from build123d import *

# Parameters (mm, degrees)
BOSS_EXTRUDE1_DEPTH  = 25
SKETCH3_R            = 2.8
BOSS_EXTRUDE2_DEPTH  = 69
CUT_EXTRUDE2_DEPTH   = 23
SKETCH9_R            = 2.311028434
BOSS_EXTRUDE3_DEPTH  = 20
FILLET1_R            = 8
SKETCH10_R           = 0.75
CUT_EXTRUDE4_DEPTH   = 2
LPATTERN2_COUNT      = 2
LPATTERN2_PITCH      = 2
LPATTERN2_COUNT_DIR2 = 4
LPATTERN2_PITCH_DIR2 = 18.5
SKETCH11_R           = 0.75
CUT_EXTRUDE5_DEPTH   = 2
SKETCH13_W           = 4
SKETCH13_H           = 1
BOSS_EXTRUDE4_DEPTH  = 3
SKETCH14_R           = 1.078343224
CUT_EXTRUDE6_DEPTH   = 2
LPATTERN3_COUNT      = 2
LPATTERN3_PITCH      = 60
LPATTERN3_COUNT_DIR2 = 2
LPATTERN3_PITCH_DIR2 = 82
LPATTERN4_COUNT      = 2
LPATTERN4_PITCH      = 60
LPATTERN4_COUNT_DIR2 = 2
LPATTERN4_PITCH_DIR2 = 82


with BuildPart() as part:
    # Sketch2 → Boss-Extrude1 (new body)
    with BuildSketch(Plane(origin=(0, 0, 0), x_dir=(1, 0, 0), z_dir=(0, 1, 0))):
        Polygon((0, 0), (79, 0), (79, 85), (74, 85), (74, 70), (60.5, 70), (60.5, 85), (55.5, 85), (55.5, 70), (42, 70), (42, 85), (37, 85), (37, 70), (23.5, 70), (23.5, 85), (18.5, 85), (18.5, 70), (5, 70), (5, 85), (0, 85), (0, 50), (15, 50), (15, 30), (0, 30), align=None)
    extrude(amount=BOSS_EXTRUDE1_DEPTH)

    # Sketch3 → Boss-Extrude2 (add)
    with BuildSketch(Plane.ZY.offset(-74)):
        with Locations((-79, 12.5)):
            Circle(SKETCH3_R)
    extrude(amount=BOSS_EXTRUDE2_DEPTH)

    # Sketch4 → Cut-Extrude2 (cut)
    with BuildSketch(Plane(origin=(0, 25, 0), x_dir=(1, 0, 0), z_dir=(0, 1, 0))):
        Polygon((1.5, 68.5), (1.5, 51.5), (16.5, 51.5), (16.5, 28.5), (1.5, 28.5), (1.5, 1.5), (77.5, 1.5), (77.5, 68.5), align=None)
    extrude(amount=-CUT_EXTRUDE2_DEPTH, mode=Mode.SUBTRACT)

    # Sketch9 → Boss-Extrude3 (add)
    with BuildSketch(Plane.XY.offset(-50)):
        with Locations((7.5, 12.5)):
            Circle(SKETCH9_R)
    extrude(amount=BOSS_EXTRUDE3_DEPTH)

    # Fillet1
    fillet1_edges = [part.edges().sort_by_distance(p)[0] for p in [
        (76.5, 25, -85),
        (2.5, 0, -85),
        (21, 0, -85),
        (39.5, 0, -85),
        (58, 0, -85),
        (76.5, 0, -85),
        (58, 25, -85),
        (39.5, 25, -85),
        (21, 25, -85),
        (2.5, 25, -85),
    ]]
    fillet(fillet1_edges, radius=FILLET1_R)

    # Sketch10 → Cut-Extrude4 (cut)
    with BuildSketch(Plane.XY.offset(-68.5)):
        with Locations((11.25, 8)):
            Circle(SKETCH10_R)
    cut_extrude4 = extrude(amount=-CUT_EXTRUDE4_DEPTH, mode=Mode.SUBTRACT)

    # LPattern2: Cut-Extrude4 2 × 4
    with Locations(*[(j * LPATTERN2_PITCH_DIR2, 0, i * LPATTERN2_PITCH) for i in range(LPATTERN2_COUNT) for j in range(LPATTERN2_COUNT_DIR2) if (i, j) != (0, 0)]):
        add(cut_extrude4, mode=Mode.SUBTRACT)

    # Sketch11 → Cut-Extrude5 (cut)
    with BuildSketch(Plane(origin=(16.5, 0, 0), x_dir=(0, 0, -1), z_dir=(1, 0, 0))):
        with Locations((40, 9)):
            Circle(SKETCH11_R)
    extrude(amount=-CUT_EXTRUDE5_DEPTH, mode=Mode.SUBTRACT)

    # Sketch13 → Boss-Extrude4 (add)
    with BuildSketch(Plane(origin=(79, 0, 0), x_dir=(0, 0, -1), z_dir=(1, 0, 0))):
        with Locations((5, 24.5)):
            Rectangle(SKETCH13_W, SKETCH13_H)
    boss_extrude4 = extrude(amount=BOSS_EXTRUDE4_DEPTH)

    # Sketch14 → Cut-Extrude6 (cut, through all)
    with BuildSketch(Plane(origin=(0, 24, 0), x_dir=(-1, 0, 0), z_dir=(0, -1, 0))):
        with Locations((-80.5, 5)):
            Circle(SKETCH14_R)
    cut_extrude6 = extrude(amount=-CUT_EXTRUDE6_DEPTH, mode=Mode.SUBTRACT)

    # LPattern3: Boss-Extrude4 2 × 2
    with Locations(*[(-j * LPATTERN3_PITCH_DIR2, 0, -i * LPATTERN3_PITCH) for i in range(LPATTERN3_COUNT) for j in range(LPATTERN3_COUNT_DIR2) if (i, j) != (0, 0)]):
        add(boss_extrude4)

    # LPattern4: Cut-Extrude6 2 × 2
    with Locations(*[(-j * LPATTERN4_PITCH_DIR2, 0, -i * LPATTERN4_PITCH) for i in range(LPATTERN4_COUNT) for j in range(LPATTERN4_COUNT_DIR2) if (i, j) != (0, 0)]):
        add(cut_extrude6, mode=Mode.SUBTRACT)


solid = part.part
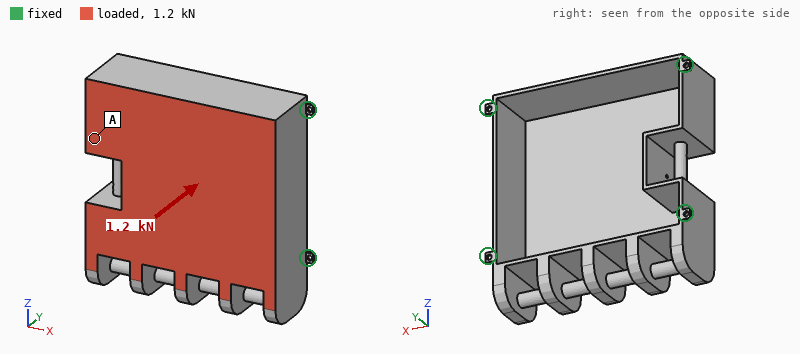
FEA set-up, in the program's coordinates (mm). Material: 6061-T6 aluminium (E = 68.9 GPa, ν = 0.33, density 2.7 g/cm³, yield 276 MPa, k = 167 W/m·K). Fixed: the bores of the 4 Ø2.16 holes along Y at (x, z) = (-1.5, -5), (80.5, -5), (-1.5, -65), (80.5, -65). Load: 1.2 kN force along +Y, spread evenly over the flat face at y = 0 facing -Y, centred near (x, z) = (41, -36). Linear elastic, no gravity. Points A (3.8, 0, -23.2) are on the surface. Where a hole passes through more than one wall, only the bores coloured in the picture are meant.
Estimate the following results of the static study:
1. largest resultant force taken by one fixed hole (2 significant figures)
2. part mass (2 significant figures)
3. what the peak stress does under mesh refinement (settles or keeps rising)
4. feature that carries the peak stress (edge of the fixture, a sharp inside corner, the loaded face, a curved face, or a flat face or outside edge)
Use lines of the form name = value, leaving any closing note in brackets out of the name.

largest resultant force taken by one fixed hole = 360 N
part mass = 86 g
what the peak stress does under mesh refinement = keeps rising
feature that carries the peak stress = edge of the fixture
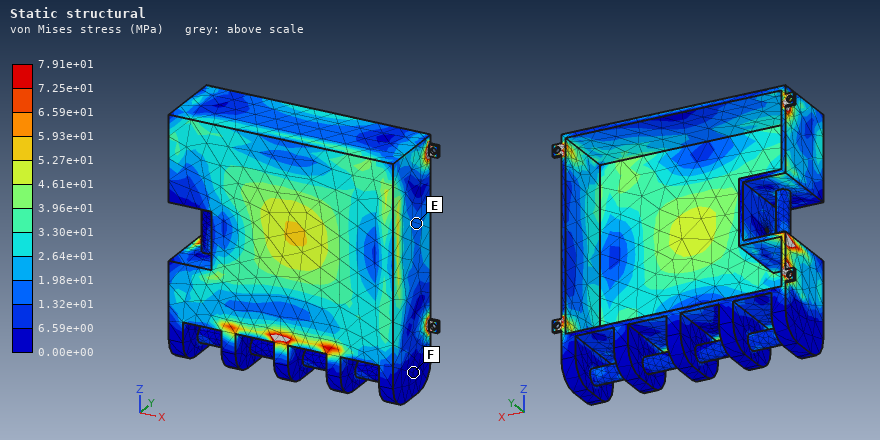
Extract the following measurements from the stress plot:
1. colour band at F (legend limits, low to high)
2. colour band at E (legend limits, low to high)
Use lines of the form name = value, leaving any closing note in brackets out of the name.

colour band at F = 0.00e+00 to 6.59e+00 MPa
colour band at E = 1.32e+01 to 1.98e+01 MPa
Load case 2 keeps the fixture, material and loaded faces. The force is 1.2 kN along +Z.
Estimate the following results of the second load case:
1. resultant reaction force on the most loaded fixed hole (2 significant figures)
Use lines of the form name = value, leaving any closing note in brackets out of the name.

resultant reaction force on the most loaded fixed hole = 590 N
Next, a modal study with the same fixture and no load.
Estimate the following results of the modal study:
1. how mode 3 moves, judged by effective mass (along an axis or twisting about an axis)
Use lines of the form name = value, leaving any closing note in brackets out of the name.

how mode 3 moves, judged by effective mass = along X
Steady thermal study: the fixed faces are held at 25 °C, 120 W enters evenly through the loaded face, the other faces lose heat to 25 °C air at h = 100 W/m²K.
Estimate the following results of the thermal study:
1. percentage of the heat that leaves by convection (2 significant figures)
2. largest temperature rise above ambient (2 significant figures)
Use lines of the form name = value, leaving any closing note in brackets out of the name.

percentage of the heat that leaves by convection = 78 %
largest temperature rise above ambient = 62 K
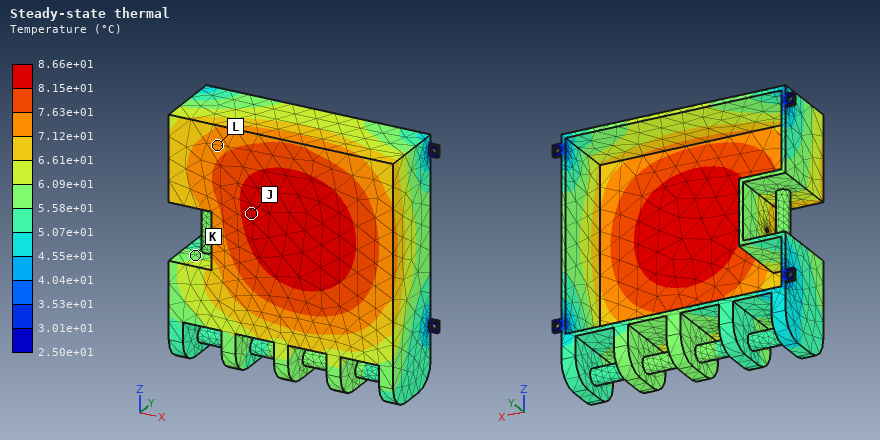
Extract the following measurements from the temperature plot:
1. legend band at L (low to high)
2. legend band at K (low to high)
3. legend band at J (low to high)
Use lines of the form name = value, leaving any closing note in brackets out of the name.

legend band at L = 7.12e+01 to 7.63e+01 °C
legend band at K = 5.58e+01 to 6.09e+01 °C
legend band at J = 8.15e+01 to 8.66e+01 °C
